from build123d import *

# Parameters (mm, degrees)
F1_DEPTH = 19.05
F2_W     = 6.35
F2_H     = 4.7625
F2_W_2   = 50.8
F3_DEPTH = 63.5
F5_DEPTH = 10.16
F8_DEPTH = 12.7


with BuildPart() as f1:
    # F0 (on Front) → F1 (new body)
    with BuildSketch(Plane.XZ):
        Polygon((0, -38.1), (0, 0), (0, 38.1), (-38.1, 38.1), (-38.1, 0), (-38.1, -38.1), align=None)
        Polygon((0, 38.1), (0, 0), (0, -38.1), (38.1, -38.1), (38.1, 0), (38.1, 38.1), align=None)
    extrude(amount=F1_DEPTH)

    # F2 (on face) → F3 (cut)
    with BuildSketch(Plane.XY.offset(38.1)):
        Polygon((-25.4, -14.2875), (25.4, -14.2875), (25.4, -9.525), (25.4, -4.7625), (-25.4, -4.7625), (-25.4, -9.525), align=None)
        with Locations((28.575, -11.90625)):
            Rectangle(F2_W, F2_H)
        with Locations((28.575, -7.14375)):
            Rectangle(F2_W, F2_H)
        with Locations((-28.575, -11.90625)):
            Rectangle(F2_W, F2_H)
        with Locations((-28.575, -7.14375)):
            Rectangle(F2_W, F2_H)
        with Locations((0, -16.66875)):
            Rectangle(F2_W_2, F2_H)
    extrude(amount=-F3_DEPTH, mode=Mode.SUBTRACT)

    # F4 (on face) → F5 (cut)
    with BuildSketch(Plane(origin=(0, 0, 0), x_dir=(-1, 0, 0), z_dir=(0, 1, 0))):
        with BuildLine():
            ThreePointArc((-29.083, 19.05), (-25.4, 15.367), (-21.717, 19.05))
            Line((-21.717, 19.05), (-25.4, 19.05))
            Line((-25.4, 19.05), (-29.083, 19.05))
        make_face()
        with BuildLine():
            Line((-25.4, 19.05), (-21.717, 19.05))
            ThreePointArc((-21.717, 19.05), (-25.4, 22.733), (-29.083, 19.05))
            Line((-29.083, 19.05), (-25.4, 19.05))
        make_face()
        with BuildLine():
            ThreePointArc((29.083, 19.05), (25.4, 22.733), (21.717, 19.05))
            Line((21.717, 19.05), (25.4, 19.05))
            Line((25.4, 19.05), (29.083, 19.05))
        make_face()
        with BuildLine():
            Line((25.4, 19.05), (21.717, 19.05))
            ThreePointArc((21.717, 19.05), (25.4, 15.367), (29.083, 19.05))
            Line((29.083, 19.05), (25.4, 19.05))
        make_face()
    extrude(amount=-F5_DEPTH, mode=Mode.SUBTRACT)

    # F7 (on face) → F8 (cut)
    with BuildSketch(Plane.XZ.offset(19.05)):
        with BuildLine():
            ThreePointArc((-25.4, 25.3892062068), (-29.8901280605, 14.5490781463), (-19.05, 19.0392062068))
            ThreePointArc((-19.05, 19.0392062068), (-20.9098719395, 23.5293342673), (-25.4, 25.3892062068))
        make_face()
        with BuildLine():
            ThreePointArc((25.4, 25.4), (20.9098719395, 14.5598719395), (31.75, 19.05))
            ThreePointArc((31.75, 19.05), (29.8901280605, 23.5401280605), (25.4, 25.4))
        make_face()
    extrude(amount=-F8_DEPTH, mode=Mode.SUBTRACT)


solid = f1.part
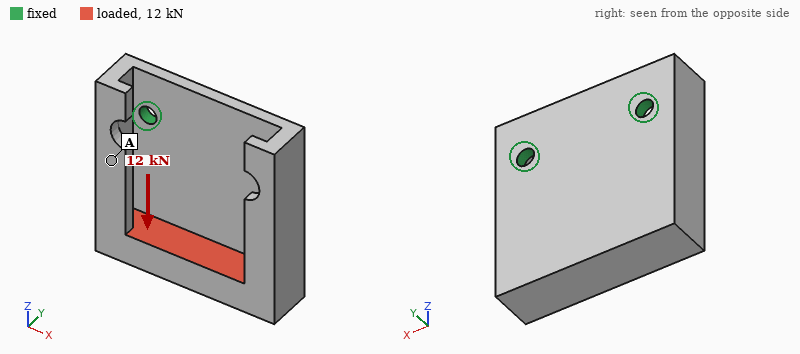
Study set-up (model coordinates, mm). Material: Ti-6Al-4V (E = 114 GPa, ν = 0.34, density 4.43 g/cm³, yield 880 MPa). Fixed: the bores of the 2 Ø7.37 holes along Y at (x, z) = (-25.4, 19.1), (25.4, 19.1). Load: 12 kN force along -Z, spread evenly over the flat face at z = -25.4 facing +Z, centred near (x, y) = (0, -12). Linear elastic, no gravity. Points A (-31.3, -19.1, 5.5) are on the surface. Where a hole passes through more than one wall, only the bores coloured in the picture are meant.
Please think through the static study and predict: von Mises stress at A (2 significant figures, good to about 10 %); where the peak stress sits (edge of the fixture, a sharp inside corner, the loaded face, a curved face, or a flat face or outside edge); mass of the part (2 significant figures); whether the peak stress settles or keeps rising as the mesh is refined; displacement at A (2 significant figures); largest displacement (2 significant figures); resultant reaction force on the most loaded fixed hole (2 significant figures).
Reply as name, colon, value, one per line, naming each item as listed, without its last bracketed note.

von Mises stress at A: 56 MPa
where the peak stress sits: edge of the fixture
mass of the part: 250 g
whether the peak stress settles or keeps rising as the mesh is refined: keeps rising
displacement at A: 0.12 mm
largest displacement: 0.39 mm
resultant reaction force on the most loaded fixed hole: 6.1 kN
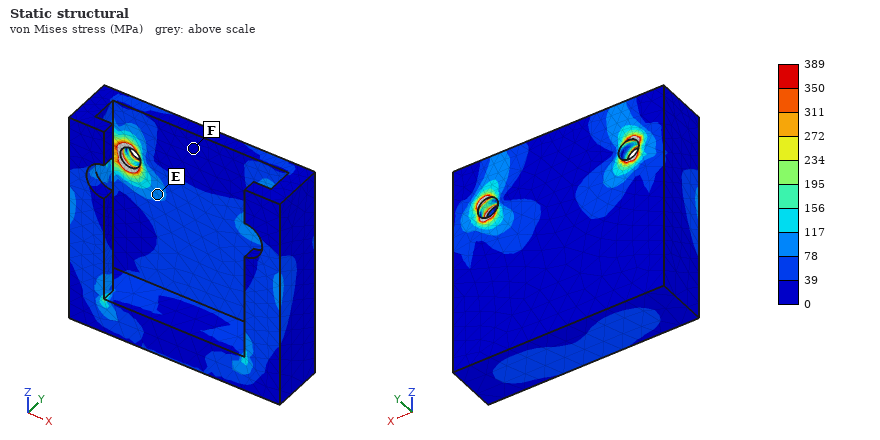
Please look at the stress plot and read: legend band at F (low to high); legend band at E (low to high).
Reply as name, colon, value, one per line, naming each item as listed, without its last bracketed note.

legend band at F: 0 to 39 MPa
legend band at E: 78 to 117 MPa
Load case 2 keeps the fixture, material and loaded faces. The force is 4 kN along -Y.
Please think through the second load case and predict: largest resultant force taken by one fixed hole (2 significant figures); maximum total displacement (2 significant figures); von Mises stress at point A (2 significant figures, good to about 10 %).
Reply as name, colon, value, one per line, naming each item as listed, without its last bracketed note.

largest resultant force taken by one fixed hole: 2.1 kN
maximum total displacement: 0.57 mm
von Mises stress at point A: 70 MPa
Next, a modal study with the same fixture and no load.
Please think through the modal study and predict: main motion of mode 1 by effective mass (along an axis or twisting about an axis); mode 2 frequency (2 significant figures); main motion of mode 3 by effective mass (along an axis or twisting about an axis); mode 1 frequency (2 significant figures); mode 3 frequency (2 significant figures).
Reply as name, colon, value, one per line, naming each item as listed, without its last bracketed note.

main motion of mode 1 by effective mass: along Y
mode 2 frequency: 2600 Hz
main motion of mode 3 by effective mass: along X
mode 1 frequency: 1300 Hz
mode 3 frequency: 5800 Hz
